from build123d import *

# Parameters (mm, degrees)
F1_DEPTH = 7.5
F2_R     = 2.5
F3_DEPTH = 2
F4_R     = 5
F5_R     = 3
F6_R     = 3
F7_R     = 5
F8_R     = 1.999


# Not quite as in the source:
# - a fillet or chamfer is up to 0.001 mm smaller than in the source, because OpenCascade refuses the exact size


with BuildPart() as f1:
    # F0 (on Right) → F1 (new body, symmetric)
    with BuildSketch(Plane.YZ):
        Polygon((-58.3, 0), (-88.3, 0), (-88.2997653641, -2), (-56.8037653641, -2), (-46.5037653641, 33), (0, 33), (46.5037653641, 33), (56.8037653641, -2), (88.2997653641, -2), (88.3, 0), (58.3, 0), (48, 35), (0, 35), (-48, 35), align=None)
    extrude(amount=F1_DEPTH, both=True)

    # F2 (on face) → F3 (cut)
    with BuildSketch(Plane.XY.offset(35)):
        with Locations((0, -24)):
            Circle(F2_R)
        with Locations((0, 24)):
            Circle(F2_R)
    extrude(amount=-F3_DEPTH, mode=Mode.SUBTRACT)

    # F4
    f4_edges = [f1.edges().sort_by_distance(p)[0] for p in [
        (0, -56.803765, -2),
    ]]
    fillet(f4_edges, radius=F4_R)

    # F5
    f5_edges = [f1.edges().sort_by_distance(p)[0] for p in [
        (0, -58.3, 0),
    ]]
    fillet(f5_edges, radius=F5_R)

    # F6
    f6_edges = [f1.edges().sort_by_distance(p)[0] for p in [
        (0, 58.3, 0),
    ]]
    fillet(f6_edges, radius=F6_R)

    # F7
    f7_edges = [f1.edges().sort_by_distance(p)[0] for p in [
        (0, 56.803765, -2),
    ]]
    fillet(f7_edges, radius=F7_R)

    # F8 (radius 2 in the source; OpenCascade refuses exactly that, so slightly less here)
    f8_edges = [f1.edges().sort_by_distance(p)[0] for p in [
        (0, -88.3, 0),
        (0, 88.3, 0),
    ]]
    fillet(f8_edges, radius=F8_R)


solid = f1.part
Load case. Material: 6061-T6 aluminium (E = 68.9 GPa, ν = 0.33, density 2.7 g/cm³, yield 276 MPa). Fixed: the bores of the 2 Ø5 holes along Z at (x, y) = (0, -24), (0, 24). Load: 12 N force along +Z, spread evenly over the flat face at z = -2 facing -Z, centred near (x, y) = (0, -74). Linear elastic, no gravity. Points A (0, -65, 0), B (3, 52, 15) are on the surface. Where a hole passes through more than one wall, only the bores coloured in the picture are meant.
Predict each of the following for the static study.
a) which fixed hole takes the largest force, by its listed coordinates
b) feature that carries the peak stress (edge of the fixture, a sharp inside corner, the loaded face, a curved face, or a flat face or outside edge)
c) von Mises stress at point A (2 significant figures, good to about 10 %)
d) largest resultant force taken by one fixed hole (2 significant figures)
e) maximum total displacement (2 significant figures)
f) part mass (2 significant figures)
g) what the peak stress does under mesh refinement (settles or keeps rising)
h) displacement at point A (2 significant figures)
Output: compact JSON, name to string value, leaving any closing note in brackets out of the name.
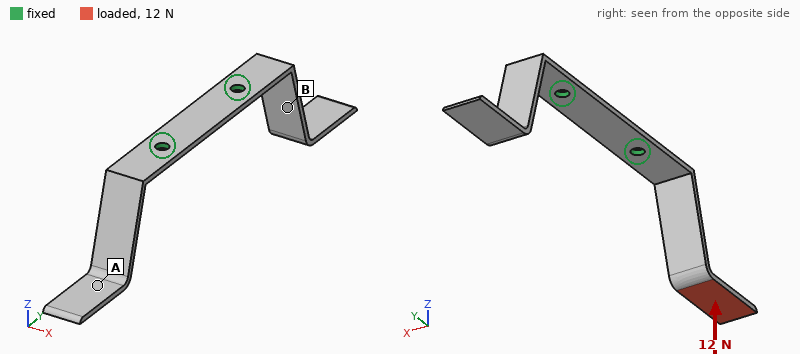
{"which fixed hole takes the largest force, by its listed coordinates": "(0, -24)", "feature that carries the peak stress": "edge of the fixture", "von Mises stress at point A": "11 MPa", "largest resultant force taken by one fixed hole": "12 N", "maximum total displacement": "1.5 mm", "part mass": "18 g", "what the peak stress does under mesh refinement": "keeps rising", "displacement at point A": "0.92 mm"}
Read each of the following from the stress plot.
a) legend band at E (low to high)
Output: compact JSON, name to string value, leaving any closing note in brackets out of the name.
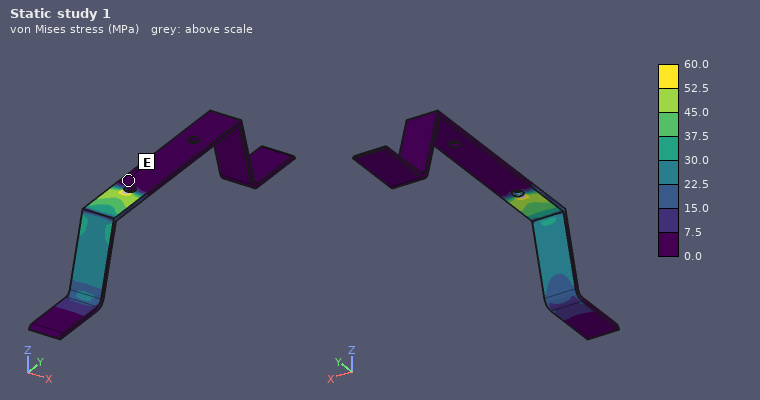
{"legend band at E": "0.0 to 7.5 MPa"}
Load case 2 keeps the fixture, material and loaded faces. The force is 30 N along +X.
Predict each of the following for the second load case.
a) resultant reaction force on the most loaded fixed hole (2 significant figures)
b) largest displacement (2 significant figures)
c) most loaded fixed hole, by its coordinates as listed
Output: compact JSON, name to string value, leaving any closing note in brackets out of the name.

{"resultant reaction force on the most loaded fixed hole": "43 N", "largest displacement": "1.2 mm", "most loaded fixed hole, by its coordinates as listed": "(0, -24)"}
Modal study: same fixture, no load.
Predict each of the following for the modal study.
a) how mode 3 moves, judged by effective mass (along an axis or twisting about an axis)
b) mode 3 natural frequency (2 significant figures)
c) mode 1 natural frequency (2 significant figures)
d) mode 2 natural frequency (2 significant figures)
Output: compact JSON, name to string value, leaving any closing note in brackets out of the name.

{"how mode 3 moves, judged by effective mass": "along X", "mode 3 natural frequency": "510 Hz", "mode 1 natural frequency": "260 Hz", "mode 2 natural frequency": "260 Hz"}
